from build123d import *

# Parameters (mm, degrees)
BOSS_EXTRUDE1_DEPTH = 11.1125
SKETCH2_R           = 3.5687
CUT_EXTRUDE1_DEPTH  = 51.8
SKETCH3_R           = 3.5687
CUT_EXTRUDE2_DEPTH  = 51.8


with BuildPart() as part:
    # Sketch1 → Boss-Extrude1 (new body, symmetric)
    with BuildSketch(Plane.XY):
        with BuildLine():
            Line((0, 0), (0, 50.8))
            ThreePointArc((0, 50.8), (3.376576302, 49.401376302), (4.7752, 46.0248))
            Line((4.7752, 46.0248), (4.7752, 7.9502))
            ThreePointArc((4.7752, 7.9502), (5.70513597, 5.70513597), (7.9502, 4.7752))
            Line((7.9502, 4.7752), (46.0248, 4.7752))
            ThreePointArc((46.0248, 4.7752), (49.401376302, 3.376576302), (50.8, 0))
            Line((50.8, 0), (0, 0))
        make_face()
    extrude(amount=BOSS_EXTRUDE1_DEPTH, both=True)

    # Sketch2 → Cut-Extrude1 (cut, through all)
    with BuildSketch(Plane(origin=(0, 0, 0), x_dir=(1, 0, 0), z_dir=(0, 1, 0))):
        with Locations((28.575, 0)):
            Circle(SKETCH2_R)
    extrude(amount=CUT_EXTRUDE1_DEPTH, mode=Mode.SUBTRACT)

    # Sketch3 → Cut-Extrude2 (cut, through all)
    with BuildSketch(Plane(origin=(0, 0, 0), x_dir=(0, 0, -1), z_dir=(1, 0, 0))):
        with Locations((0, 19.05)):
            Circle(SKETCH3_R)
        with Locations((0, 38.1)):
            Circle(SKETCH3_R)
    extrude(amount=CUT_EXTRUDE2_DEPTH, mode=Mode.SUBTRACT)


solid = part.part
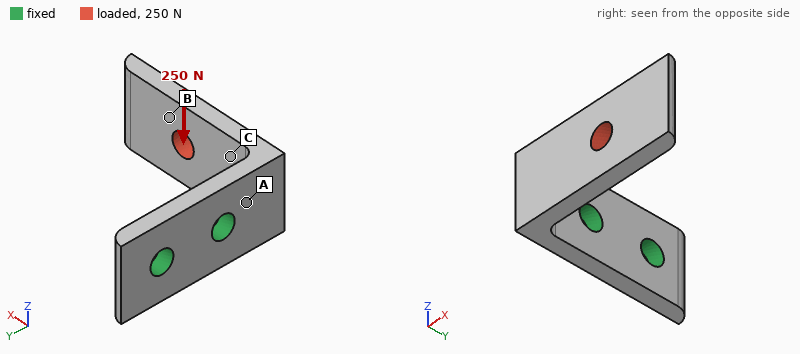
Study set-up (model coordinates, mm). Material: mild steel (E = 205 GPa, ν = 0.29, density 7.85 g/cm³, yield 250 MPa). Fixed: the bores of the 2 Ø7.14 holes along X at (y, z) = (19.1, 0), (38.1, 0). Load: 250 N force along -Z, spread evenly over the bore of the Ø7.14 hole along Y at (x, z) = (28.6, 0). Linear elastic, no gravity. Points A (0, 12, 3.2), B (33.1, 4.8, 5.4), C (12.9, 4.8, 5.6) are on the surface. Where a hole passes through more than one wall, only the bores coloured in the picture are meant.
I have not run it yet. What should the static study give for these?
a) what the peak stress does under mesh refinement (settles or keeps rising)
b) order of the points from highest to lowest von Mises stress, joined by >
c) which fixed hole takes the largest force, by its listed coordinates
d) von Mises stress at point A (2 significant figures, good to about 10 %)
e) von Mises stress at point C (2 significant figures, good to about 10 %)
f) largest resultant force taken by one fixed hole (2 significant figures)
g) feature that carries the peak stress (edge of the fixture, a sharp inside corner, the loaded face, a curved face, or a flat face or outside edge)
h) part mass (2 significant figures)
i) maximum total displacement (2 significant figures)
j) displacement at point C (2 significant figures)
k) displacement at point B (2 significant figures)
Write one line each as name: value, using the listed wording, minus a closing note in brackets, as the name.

what the peak stress does under mesh refinement: keeps rising
order of the points from highest to lowest von Mises stress, joined by >: A > C > B
which fixed hole takes the largest force, by its listed coordinates: (19.1, 0)
von Mises stress at point A: 45 MPa
von Mises stress at point C: 14 MPa
largest resultant force taken by one fixed hole: 340 N
feature that carries the peak stress: edge of the fixture
part mass: 75 g
maximum total displacement: 60 µm
displacement at point C: 15 µm
displacement at point B: 39 µm
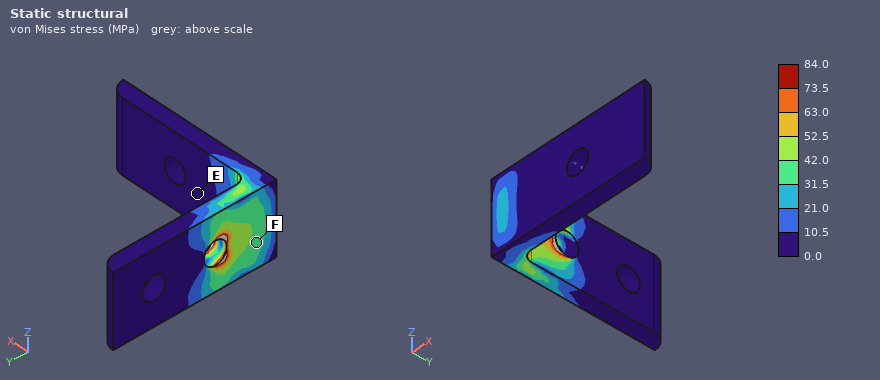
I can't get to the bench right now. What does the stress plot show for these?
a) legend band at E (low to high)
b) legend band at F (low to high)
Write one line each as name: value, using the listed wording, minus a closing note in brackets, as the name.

legend band at E: 0.0 to 10.5 MPa
legend band at F: 31.5 to 42.0 MPa
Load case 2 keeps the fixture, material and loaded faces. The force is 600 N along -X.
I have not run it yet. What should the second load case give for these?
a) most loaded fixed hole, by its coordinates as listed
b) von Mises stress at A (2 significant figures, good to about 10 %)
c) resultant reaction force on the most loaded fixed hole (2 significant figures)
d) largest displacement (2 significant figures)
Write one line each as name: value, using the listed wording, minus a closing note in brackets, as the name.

most loaded fixed hole, by its coordinates as listed: (19.1, 0)
von Mises stress at A: 67 MPa
resultant reaction force on the most loaded fixed hole: 660 N
largest displacement: 79 µm
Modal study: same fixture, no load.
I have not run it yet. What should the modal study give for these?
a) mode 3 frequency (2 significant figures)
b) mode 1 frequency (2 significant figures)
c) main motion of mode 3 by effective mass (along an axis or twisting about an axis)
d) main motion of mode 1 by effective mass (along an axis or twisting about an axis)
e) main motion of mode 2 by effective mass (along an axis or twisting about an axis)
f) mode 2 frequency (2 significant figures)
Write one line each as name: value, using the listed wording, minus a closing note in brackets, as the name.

mode 3 frequency: 5600 Hz
mode 1 frequency: 1300 Hz
main motion of mode 3 by effective mass: along X
main motion of mode 1 by effective mass: along Y
main motion of mode 2 by effective mass: along Z
mode 2 frequency: 2100 Hz
